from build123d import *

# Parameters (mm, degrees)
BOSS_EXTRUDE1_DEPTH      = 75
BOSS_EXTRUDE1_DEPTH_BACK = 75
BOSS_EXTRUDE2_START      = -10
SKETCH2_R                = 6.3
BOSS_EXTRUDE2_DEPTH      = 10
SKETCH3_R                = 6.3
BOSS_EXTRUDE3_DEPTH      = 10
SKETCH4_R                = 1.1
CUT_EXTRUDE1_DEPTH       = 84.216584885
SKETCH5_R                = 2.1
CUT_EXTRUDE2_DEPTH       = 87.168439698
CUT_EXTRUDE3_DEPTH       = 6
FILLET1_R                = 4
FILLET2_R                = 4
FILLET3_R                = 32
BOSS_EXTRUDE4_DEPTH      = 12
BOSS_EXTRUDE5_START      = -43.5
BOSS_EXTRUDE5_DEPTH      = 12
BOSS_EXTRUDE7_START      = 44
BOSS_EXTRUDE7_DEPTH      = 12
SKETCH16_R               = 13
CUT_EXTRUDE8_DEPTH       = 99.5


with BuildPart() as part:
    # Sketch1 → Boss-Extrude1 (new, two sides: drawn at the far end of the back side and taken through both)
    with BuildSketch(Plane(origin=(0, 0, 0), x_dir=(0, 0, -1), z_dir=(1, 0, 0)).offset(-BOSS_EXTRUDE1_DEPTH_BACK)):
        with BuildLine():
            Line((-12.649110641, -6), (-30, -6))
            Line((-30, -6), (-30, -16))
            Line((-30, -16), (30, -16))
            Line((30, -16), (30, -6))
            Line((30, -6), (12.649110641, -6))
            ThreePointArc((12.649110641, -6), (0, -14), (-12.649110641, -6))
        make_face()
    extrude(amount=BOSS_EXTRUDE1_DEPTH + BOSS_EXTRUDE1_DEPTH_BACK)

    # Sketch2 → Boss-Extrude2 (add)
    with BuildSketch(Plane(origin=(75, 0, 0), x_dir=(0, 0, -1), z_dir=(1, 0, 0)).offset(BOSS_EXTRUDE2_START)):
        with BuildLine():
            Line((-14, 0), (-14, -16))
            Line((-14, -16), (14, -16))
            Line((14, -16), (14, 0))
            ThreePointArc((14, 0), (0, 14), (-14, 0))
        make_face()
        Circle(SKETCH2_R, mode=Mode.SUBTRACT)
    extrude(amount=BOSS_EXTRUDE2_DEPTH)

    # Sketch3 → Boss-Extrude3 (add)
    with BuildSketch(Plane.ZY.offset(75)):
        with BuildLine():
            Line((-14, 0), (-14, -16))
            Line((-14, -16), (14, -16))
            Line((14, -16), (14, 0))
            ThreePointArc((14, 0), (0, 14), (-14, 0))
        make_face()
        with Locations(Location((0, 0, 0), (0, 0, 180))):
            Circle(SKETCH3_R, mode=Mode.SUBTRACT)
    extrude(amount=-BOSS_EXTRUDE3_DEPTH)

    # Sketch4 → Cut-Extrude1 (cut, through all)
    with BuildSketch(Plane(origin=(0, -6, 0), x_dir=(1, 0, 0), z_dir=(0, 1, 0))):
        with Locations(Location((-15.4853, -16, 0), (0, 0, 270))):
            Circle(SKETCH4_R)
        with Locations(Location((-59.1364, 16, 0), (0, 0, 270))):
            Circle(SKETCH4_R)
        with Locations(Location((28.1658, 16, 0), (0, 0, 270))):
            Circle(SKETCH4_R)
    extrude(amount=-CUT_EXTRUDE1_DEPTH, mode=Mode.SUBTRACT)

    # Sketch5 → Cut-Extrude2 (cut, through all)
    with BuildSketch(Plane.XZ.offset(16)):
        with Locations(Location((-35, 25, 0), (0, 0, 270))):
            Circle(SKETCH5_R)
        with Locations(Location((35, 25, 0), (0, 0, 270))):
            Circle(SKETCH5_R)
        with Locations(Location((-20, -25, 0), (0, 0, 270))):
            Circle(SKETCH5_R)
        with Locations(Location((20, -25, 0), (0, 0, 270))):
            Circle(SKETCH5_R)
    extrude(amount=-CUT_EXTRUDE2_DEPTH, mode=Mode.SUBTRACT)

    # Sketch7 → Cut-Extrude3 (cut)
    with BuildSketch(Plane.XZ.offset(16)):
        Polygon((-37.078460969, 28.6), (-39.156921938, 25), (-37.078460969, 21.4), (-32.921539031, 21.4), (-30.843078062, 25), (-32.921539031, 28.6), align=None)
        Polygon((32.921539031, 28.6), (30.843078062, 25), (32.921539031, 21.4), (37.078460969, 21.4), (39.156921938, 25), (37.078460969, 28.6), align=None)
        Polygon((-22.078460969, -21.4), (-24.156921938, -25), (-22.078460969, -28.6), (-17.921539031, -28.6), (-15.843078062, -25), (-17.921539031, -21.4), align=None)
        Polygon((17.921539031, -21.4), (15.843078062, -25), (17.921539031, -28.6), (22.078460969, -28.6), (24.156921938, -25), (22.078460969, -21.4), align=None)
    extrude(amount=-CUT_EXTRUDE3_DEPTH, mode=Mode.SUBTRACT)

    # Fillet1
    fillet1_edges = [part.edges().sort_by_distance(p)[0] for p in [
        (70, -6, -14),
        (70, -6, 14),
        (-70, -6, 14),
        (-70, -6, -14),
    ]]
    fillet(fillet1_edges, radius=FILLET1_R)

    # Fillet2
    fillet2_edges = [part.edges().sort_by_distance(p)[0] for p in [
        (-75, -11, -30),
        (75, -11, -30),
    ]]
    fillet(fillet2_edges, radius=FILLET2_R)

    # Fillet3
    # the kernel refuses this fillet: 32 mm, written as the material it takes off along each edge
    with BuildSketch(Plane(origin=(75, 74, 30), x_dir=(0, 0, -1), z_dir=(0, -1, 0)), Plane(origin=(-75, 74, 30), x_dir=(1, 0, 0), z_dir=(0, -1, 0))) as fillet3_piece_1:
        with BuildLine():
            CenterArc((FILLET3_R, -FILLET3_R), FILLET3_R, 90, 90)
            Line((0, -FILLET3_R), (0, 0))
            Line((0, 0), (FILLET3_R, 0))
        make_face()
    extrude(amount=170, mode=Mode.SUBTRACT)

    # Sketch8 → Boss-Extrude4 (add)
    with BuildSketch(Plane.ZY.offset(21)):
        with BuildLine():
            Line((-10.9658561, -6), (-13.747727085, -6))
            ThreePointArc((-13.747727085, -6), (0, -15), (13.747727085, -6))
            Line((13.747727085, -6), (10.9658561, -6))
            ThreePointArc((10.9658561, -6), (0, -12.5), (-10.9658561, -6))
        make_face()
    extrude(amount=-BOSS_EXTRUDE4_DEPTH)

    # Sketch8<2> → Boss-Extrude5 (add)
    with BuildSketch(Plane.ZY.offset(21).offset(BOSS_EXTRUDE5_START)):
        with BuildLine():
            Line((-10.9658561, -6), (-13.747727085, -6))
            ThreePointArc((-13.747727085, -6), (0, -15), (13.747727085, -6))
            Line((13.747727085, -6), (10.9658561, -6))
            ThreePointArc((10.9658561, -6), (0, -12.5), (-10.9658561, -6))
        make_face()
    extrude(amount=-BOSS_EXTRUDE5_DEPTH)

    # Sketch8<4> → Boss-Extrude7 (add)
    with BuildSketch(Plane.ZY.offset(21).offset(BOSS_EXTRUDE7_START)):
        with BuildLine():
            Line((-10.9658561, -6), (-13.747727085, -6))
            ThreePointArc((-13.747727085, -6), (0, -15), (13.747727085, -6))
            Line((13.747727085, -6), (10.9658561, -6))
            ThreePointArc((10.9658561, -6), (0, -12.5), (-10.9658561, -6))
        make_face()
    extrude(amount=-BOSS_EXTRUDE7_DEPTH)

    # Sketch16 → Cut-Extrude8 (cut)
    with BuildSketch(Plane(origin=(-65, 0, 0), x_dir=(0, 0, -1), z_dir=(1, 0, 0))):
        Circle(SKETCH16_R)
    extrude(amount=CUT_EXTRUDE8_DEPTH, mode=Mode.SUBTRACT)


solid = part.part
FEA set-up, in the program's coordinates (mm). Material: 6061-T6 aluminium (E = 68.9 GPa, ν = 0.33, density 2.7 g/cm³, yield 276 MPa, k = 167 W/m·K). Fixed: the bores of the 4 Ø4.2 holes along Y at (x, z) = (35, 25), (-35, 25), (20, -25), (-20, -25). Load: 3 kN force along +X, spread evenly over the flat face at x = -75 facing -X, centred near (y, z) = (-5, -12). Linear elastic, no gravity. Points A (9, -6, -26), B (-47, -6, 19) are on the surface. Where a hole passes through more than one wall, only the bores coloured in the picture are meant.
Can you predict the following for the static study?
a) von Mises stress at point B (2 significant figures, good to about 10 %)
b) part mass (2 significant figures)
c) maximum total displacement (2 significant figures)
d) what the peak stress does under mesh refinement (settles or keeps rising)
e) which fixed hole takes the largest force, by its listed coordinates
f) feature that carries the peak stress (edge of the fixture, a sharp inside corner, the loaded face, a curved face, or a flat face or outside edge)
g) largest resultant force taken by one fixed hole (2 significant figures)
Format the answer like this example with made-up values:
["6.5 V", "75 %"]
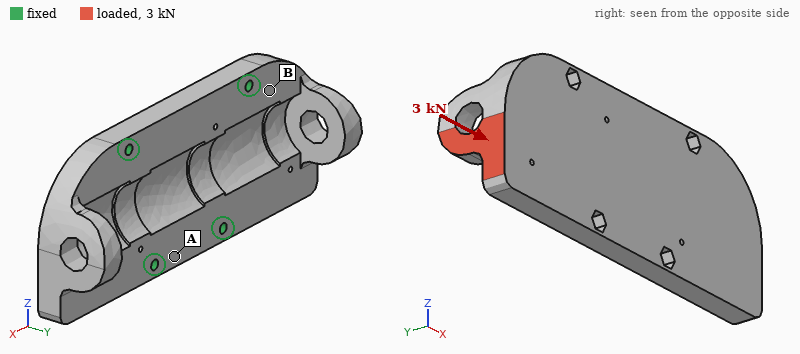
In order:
["30 MPa", "200 g", "0.18 mm", "keeps rising", "(-20, -25)", "edge of the fixture", "2.1 kN"]
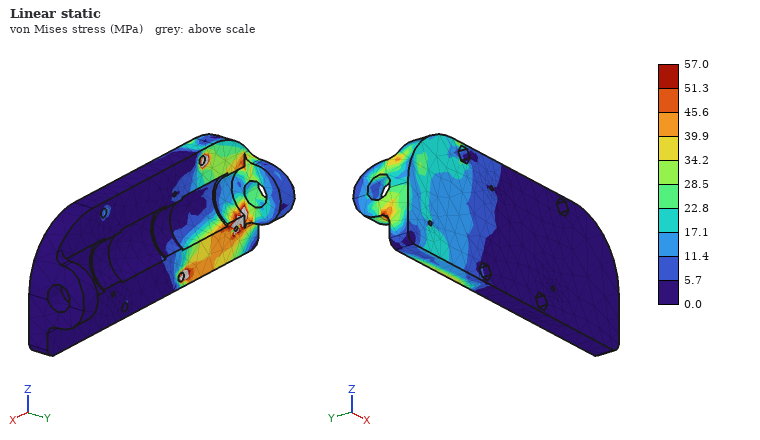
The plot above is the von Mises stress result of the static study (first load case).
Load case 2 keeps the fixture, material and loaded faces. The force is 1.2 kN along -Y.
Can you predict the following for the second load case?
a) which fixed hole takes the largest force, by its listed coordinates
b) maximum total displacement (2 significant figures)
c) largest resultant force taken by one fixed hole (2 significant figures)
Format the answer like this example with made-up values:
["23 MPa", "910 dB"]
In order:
["(-20, -25)", "0.38 mm", "2.3 kN"]
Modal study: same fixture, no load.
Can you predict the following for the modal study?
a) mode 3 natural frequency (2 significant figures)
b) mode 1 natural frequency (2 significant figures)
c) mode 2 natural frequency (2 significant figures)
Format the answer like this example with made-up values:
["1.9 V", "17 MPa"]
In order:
["4700 Hz", "2100 Hz", "2100 Hz"]
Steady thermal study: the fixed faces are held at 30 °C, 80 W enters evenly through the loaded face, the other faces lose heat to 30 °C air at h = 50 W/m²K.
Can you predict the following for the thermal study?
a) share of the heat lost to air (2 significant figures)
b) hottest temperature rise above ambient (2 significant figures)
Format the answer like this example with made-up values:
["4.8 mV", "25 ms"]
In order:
["20 %", "72 K"]
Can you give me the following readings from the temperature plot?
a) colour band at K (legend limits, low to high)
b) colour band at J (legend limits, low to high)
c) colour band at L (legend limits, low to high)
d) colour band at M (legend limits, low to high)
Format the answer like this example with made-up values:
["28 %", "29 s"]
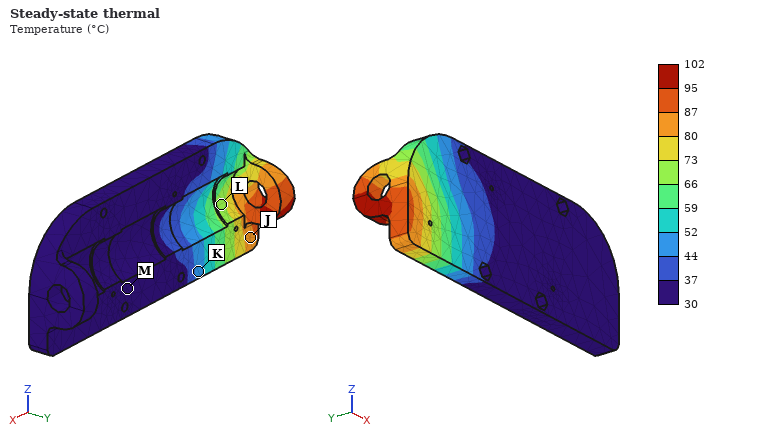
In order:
["44 to 52 °C", "80 to 87 °C", "66 to 73 °C", "30 to 37 °C"]
